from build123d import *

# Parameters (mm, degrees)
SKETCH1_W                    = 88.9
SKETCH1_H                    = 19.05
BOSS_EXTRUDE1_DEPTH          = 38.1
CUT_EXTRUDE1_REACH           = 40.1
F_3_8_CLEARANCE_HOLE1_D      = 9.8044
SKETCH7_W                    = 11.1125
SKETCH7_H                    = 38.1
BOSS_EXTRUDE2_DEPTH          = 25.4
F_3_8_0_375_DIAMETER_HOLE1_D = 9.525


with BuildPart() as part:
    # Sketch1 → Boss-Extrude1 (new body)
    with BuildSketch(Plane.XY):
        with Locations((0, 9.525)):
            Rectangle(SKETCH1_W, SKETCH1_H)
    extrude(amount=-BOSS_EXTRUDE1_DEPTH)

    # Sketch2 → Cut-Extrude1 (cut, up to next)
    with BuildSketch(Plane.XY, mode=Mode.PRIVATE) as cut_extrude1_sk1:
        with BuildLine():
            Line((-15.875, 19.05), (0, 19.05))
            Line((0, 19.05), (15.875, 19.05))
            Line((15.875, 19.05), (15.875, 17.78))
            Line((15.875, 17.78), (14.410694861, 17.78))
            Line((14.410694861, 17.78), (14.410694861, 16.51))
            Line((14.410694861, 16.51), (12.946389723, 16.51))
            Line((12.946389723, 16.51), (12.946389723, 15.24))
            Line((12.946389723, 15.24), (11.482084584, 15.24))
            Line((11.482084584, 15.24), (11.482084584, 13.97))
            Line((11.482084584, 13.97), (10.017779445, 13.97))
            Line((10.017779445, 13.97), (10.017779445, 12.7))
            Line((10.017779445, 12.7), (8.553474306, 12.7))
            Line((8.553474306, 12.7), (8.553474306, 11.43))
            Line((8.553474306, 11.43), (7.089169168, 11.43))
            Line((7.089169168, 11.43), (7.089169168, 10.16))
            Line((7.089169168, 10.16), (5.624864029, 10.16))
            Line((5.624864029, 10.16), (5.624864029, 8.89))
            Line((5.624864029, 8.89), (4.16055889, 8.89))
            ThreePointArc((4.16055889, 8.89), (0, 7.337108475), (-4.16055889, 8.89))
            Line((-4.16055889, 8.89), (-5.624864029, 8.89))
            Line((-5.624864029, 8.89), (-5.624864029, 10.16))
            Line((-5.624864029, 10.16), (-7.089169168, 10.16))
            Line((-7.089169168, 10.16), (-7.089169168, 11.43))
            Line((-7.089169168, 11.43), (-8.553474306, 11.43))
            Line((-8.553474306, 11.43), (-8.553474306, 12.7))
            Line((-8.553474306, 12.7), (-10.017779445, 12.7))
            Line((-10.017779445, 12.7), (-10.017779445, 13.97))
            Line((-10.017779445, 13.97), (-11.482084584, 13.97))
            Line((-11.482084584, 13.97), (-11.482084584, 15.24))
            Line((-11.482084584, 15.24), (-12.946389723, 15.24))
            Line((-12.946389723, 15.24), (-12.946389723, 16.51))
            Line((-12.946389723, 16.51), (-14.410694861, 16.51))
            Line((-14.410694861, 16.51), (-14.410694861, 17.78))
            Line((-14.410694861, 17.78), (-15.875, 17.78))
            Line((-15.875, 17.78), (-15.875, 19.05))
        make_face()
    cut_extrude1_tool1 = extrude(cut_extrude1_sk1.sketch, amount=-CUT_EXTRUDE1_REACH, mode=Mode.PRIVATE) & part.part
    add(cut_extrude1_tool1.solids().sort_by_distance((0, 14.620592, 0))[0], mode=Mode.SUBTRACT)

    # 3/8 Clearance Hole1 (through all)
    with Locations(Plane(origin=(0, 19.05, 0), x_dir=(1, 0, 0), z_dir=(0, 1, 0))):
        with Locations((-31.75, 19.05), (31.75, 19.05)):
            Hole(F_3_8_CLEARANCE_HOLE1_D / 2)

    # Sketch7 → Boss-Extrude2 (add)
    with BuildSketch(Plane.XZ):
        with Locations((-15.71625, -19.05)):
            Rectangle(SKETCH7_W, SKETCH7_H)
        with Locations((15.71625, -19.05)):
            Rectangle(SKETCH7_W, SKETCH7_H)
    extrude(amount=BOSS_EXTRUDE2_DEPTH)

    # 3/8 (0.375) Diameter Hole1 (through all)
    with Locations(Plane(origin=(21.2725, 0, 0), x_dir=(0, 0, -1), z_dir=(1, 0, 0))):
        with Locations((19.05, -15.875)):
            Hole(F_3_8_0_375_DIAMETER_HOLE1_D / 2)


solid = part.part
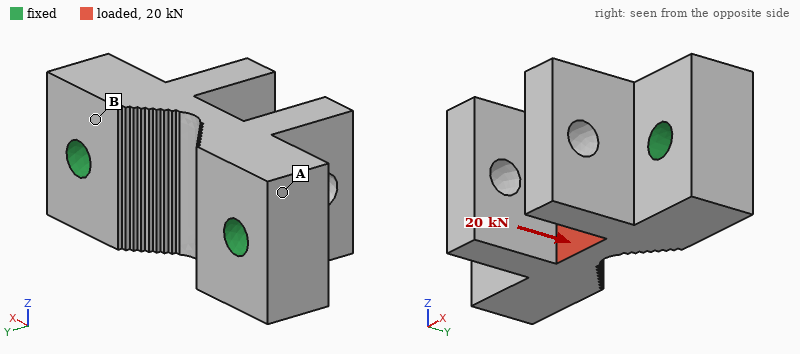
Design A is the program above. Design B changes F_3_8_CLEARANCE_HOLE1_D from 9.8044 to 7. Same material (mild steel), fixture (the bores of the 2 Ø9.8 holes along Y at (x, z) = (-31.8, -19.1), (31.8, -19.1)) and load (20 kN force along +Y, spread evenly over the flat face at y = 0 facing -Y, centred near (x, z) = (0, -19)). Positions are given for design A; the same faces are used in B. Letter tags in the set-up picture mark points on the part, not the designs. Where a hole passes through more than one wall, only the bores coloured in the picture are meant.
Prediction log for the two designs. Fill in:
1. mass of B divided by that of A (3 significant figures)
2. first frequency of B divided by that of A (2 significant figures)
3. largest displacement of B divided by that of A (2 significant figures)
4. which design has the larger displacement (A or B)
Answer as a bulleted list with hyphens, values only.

- 1.02
- 0.96
- 1.2
- B
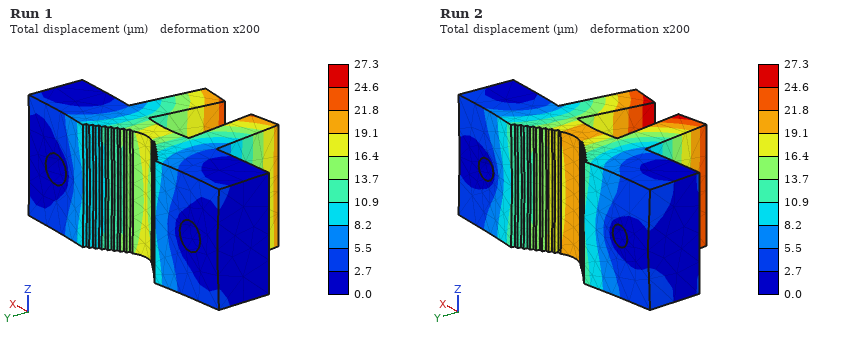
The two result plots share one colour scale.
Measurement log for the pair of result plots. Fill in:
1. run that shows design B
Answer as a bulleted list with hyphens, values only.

- Run 2
